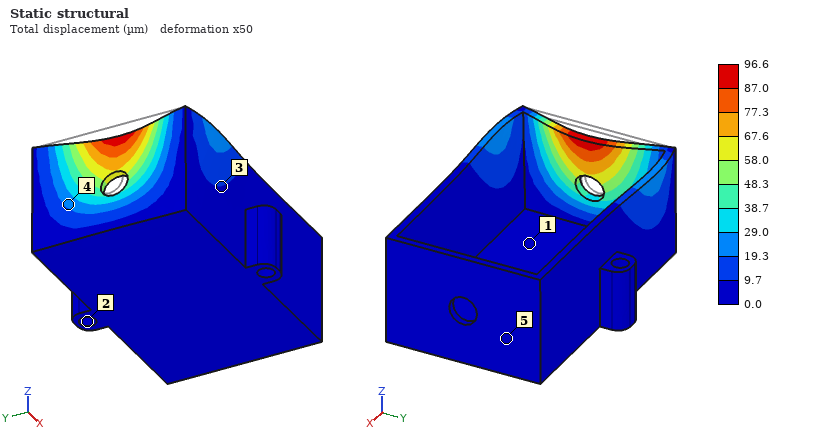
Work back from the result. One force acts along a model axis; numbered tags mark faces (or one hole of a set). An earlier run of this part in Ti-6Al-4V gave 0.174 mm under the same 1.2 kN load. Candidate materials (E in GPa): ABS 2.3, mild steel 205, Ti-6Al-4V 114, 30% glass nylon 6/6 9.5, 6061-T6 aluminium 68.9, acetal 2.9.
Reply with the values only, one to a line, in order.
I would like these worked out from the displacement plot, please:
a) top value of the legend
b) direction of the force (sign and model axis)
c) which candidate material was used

96.6 µm
+X
mild steel
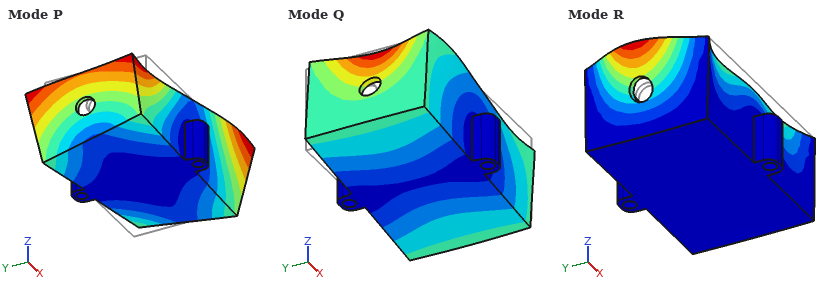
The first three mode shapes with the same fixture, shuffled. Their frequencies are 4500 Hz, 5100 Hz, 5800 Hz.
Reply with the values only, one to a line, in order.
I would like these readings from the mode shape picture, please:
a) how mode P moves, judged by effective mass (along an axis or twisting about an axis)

twisting about Z
